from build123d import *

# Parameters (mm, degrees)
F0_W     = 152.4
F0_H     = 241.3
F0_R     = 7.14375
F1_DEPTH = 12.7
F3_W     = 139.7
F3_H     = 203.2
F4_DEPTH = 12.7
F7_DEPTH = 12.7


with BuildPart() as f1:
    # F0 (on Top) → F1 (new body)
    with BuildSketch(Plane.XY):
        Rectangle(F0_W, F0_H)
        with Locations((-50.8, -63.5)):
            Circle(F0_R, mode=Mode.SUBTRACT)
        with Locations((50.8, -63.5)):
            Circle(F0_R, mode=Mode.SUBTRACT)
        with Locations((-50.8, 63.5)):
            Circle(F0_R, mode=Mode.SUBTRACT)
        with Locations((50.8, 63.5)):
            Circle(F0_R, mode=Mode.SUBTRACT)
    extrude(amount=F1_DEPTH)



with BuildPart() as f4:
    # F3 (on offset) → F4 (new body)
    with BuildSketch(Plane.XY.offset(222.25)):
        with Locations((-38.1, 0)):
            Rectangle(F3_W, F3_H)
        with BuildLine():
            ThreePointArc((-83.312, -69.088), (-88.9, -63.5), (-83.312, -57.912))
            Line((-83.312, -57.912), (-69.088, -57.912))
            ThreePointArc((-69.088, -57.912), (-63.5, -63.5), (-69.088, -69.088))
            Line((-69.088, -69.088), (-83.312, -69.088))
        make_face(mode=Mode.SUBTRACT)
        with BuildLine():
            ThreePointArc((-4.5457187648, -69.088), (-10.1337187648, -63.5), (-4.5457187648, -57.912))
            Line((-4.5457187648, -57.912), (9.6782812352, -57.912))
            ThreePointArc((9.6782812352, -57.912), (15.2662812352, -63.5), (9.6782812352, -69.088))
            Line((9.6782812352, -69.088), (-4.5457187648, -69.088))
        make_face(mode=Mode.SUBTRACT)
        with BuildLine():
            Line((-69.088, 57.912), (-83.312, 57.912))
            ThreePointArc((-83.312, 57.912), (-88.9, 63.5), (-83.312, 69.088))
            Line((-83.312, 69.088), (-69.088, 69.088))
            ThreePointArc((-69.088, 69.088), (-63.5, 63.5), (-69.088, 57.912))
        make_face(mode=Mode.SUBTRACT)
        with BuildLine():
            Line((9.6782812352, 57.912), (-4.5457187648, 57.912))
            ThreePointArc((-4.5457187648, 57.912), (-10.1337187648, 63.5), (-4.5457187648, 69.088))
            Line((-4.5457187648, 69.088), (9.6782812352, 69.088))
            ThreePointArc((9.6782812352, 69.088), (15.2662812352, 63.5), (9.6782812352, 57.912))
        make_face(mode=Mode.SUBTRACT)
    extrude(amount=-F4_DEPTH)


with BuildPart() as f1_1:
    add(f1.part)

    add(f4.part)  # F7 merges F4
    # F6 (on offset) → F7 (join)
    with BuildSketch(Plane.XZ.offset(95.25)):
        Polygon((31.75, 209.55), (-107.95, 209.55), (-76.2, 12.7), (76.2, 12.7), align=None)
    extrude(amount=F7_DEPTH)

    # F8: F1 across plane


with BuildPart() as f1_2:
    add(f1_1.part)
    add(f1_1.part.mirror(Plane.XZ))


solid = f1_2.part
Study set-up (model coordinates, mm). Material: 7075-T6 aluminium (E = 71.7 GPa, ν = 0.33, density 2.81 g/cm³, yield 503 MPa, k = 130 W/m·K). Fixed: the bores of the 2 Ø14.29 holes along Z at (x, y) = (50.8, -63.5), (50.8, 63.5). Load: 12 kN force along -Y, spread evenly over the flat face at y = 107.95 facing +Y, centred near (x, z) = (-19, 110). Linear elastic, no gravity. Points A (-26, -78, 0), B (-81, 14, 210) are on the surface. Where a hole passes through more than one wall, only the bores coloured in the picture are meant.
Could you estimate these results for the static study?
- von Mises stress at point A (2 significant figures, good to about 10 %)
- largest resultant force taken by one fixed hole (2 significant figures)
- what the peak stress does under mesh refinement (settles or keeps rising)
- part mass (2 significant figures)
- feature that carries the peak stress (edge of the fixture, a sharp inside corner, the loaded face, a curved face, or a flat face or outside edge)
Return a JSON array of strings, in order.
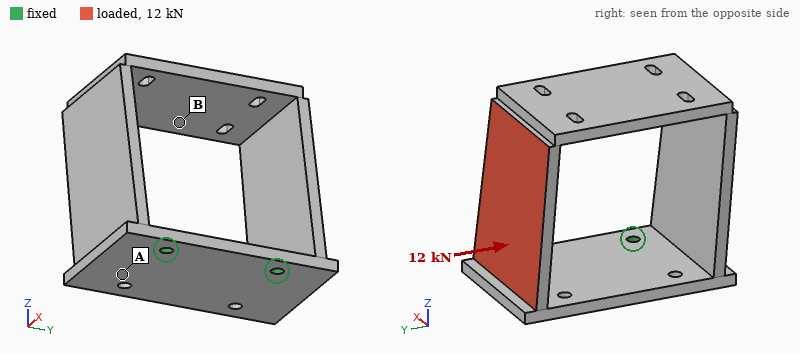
["66 MPa", "10 kN", "keeps rising", "4.3 kg", "edge of the fixture"]
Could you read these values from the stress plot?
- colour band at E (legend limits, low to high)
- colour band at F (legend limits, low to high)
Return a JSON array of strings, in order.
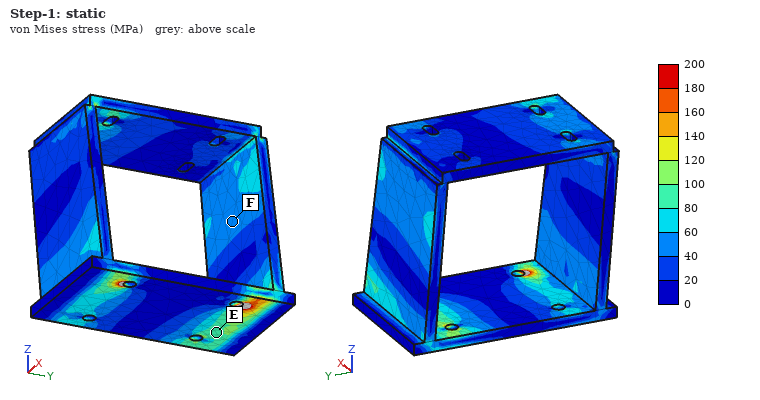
["80 to 100 MPa", "40 to 60 MPa"]
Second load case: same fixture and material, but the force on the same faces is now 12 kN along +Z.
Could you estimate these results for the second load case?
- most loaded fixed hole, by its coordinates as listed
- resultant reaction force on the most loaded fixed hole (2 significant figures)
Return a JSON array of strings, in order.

["(50.8, 63.5)", "13 kN"]
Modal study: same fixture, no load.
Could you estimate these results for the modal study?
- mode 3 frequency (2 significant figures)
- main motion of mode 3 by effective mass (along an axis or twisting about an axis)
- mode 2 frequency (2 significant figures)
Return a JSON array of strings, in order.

["360 Hz", "twisting about Z", "170 Hz"]
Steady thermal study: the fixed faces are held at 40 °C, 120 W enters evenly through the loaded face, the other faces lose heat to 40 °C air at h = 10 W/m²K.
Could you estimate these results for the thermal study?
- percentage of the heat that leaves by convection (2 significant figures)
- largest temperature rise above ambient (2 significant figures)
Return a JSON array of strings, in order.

["36 %", "43 K"]
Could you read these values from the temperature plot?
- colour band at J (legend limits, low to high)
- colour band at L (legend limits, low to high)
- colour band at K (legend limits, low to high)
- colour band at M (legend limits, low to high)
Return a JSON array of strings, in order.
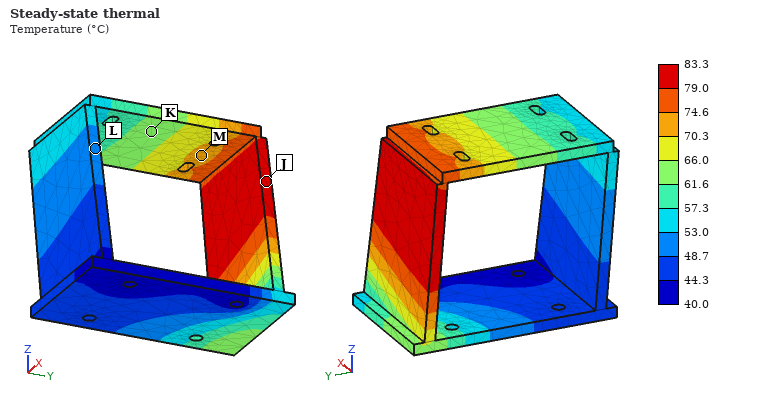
["79.0 to 83.3 °C", "48.7 to 53.0 °C", "61.6 to 66.0 °C", "70.3 to 74.6 °C"]
